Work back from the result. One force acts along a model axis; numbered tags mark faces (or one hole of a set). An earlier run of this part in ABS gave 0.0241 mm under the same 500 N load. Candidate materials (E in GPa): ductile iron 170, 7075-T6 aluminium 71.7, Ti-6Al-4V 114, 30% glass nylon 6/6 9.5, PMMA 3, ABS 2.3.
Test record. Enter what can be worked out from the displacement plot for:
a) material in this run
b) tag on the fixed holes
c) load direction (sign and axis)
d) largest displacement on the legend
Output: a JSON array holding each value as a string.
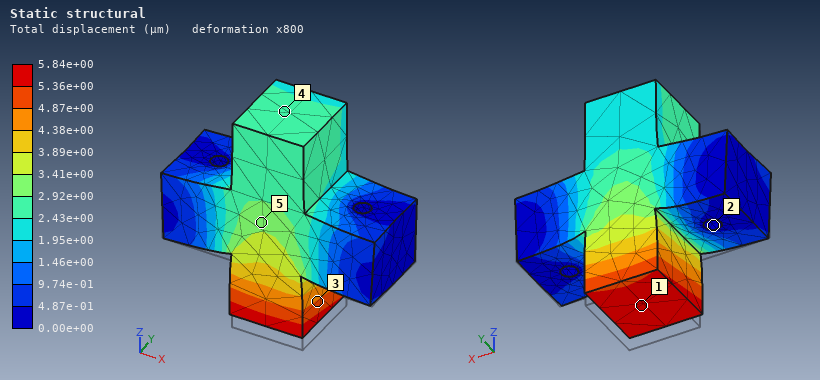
["30% glass nylon 6/6", "2", "+Z", "5.84e+00 µm"]
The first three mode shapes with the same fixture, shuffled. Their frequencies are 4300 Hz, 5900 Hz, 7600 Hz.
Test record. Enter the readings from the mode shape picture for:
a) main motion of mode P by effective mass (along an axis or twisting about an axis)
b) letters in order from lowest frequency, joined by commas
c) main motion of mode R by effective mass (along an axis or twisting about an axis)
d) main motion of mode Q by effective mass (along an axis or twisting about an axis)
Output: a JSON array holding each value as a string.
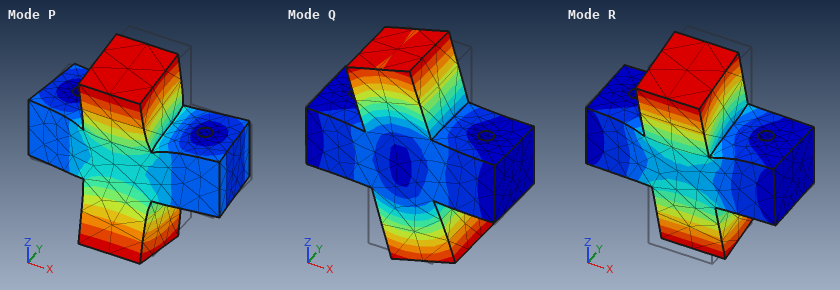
["along Y", "R, P, Q", "twisting about X", "twisting about Y"]
